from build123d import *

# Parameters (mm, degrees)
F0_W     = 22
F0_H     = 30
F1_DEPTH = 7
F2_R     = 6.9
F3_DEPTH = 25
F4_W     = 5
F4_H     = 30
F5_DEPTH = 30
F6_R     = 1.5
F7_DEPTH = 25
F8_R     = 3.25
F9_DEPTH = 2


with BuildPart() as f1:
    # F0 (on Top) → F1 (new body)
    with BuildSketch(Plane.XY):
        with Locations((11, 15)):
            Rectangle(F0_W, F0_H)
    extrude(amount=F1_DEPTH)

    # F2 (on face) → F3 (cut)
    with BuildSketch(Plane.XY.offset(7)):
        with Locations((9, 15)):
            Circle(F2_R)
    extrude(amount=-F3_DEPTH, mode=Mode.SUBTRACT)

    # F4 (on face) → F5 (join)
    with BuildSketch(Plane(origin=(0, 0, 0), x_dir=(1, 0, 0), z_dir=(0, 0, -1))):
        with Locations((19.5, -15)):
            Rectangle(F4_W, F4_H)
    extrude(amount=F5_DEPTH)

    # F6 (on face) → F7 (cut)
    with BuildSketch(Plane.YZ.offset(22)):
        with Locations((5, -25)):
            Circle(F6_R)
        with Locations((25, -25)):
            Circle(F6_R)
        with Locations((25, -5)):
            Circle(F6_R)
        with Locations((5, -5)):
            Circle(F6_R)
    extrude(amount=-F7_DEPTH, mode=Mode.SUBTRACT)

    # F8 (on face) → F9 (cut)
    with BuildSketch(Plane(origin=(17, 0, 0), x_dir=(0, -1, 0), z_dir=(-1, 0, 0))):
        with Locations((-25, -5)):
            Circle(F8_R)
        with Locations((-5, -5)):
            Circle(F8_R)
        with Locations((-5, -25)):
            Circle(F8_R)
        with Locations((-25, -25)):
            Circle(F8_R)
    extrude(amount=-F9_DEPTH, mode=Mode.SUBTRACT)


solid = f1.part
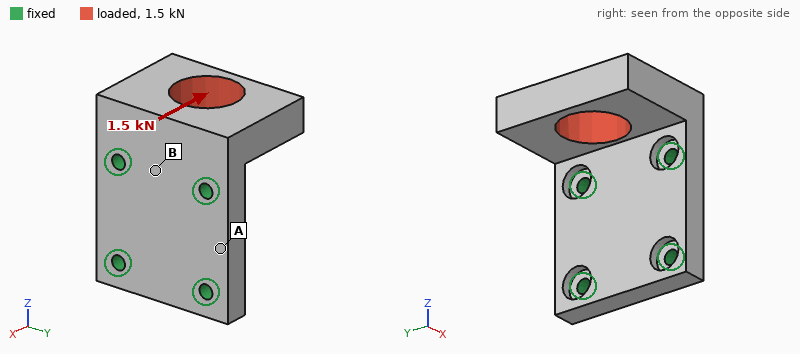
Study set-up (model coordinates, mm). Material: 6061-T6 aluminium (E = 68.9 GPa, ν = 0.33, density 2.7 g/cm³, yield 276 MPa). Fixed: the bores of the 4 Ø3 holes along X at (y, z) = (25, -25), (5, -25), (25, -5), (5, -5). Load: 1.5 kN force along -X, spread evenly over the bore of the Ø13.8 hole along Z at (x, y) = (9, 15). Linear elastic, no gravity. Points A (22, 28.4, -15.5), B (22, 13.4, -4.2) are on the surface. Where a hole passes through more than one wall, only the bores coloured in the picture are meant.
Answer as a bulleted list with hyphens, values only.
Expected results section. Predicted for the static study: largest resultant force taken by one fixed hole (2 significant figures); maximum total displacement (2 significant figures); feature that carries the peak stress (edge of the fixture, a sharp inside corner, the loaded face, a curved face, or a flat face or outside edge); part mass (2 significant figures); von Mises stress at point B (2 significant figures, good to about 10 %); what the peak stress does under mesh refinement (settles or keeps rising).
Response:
- 970 N
- 0.11 mm
- edge of the fixture
- 21 g
- 53 MPa
- keeps rising
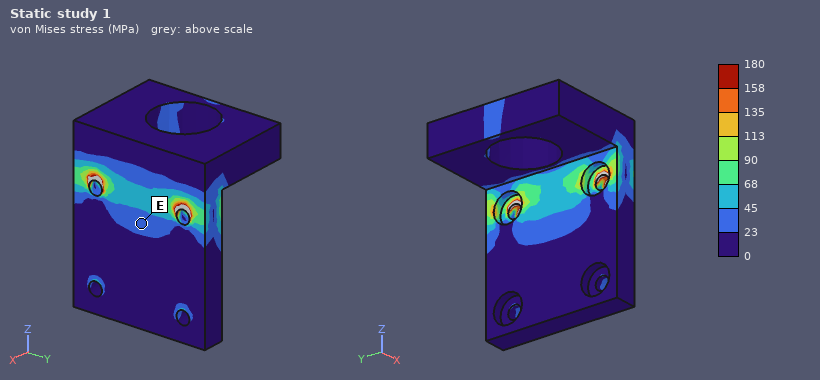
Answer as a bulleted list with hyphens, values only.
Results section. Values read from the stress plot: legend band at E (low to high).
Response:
- 23 to 45 MPa
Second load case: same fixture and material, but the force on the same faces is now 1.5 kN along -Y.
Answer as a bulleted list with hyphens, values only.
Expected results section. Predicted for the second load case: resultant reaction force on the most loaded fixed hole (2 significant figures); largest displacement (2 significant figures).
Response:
- 1.2 kN
- 56 µm
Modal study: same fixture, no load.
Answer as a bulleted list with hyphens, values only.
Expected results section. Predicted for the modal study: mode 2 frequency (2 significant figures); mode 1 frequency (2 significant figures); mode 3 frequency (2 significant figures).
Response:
- 10000 Hz
- 5300 Hz
- 15 kHz
